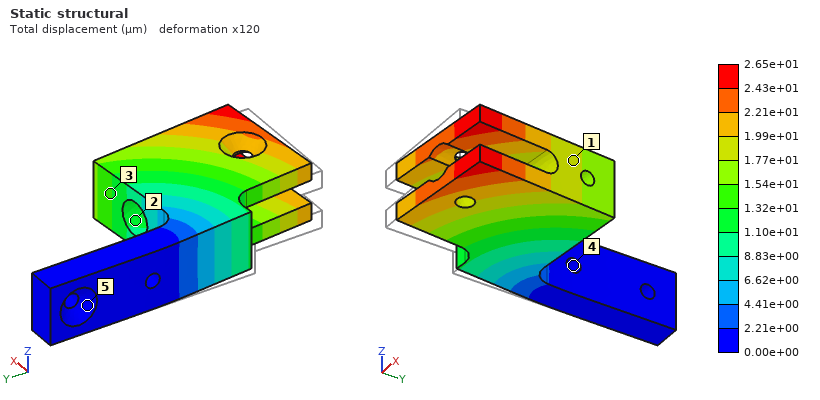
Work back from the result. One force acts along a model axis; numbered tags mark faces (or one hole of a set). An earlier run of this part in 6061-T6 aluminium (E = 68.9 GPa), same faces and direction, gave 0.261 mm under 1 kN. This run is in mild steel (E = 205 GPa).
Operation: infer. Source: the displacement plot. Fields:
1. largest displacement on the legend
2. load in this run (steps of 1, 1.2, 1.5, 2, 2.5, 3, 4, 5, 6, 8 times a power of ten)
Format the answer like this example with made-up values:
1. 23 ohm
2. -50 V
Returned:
1. 2.65e+01 µm
2. 300 N
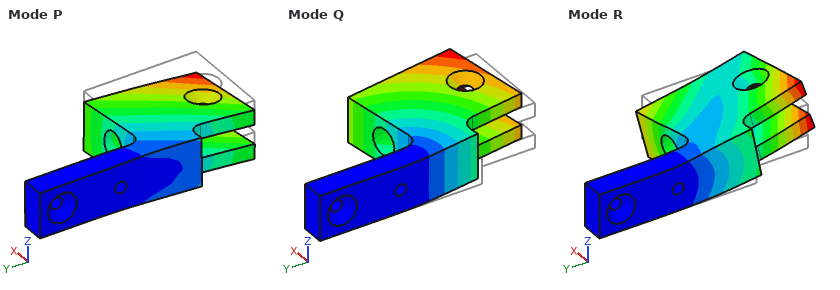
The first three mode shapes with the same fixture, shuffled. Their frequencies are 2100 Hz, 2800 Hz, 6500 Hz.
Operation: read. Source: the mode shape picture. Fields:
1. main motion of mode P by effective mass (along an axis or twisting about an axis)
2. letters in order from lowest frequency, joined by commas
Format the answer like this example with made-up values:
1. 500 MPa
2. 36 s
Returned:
1. along Z
2. Q, P, R
